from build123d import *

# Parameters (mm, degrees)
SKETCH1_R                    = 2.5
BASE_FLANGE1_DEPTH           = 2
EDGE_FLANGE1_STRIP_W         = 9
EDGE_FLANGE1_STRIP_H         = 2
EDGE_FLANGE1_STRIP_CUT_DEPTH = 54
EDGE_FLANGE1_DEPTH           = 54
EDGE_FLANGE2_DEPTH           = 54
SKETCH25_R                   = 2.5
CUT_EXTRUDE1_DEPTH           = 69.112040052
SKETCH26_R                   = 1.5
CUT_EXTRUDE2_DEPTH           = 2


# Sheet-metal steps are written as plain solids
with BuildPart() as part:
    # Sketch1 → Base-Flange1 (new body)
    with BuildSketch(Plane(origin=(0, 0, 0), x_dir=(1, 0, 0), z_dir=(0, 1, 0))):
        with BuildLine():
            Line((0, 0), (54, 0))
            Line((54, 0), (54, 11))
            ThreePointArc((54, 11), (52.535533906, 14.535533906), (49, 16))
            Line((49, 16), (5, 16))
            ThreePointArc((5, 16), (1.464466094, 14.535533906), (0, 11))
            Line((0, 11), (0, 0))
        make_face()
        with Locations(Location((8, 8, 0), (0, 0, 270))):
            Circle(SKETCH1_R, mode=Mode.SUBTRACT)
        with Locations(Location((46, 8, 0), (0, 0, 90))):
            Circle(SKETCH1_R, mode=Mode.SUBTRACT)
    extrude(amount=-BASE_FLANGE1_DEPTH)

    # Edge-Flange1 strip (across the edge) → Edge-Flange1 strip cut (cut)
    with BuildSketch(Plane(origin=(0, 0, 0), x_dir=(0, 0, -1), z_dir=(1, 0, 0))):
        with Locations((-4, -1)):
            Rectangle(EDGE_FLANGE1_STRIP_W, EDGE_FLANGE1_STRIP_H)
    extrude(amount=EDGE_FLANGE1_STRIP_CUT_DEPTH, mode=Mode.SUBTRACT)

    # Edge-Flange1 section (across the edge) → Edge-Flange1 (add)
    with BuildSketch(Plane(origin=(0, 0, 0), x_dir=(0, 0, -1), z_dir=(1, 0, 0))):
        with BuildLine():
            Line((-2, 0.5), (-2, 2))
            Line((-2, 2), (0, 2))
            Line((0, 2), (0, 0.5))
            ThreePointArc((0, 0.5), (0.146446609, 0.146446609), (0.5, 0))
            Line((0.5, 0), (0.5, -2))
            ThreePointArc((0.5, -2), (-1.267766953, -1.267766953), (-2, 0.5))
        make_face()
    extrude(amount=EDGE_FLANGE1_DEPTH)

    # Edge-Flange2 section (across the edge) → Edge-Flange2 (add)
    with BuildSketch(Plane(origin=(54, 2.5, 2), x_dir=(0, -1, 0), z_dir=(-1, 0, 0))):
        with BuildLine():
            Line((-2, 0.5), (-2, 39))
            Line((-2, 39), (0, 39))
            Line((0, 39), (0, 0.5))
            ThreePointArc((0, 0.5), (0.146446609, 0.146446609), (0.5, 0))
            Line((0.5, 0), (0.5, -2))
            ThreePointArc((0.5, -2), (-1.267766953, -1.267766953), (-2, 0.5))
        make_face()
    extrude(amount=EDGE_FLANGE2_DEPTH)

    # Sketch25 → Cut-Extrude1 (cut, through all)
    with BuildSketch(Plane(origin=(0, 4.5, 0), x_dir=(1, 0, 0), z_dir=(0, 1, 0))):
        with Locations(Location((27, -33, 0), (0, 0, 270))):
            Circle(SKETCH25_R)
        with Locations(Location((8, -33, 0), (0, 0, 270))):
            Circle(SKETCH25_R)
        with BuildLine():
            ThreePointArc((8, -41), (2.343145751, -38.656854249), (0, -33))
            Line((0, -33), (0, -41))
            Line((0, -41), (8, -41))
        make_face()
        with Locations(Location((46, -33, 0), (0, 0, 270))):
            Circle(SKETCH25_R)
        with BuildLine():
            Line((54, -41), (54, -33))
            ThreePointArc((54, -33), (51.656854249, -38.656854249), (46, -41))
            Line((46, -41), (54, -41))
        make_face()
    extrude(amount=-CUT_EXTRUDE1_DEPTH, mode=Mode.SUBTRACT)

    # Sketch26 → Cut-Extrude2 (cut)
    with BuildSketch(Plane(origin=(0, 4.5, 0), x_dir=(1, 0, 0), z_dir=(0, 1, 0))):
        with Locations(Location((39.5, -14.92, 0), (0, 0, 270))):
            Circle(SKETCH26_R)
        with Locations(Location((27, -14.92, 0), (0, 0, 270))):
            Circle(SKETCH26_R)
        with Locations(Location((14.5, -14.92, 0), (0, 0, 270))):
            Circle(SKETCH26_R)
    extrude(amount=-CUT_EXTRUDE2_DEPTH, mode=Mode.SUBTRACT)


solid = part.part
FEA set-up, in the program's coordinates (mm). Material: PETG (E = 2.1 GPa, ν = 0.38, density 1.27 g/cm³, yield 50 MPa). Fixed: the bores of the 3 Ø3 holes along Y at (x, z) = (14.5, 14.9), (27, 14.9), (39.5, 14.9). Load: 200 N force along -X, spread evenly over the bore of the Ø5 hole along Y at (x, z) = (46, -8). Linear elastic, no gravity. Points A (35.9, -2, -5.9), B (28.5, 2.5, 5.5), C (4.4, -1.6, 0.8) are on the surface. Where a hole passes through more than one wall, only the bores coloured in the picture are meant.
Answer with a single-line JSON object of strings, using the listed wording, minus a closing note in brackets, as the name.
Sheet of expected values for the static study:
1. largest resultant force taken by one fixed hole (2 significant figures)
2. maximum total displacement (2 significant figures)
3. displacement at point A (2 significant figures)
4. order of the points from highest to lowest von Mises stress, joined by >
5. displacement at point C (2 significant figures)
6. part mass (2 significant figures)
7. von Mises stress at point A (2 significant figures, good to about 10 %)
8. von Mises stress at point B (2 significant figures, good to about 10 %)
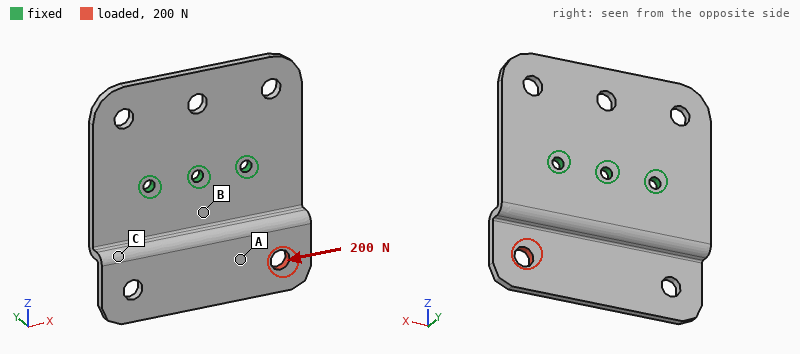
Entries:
{"largest resultant force taken by one fixed hole": "190 N", "maximum total displacement": "0.50 mm", "displacement at point A": "0.24 mm", "order of the points from highest to lowest von Mises stress, joined by >": "B > A > C", "displacement at point C": "0.35 mm", "part mass": "7.9 g", "von Mises stress at point A": "5.4 MPa", "von Mises stress at point B": "9.0 MPa"}
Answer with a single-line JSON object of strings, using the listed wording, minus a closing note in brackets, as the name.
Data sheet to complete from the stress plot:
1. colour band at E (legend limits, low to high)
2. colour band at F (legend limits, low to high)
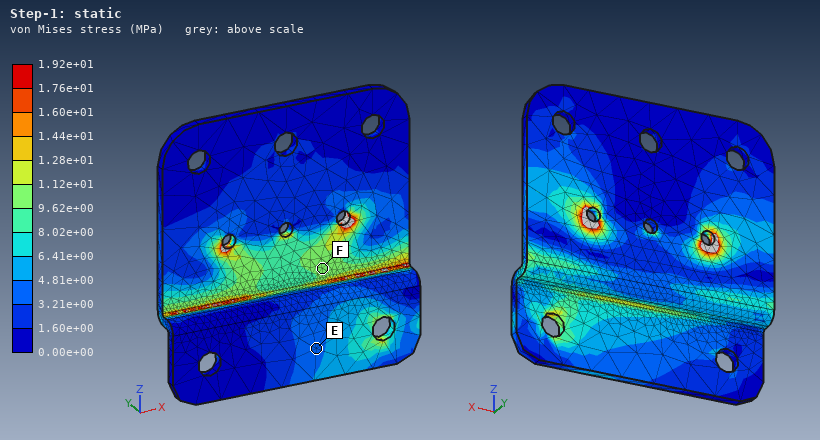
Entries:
{"colour band at E": "3.21e+00 to 4.81e+00 MPa", "colour band at F": "9.62e+00 to 1.12e+01 MPa"}
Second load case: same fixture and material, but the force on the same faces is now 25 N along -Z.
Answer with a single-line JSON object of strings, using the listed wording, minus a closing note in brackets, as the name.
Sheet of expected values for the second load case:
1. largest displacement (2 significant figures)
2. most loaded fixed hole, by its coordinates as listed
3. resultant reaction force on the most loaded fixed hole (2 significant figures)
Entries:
{"largest displacement": "0.81 mm", "most loaded fixed hole, by its coordinates as listed": "(39.5, 14.9)", "resultant reaction force on the most loaded fixed hole": "28 N"}
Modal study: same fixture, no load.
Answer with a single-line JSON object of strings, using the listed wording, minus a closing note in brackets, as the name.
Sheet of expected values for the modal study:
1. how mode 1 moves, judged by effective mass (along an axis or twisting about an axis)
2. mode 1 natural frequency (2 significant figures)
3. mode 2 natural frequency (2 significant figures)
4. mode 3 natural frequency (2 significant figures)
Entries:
{"how mode 1 moves, judged by effective mass": "along Y", "mode 1 natural frequency": "420 Hz", "mode 2 natural frequency": "670 Hz", "mode 3 natural frequency": "670 Hz"}
